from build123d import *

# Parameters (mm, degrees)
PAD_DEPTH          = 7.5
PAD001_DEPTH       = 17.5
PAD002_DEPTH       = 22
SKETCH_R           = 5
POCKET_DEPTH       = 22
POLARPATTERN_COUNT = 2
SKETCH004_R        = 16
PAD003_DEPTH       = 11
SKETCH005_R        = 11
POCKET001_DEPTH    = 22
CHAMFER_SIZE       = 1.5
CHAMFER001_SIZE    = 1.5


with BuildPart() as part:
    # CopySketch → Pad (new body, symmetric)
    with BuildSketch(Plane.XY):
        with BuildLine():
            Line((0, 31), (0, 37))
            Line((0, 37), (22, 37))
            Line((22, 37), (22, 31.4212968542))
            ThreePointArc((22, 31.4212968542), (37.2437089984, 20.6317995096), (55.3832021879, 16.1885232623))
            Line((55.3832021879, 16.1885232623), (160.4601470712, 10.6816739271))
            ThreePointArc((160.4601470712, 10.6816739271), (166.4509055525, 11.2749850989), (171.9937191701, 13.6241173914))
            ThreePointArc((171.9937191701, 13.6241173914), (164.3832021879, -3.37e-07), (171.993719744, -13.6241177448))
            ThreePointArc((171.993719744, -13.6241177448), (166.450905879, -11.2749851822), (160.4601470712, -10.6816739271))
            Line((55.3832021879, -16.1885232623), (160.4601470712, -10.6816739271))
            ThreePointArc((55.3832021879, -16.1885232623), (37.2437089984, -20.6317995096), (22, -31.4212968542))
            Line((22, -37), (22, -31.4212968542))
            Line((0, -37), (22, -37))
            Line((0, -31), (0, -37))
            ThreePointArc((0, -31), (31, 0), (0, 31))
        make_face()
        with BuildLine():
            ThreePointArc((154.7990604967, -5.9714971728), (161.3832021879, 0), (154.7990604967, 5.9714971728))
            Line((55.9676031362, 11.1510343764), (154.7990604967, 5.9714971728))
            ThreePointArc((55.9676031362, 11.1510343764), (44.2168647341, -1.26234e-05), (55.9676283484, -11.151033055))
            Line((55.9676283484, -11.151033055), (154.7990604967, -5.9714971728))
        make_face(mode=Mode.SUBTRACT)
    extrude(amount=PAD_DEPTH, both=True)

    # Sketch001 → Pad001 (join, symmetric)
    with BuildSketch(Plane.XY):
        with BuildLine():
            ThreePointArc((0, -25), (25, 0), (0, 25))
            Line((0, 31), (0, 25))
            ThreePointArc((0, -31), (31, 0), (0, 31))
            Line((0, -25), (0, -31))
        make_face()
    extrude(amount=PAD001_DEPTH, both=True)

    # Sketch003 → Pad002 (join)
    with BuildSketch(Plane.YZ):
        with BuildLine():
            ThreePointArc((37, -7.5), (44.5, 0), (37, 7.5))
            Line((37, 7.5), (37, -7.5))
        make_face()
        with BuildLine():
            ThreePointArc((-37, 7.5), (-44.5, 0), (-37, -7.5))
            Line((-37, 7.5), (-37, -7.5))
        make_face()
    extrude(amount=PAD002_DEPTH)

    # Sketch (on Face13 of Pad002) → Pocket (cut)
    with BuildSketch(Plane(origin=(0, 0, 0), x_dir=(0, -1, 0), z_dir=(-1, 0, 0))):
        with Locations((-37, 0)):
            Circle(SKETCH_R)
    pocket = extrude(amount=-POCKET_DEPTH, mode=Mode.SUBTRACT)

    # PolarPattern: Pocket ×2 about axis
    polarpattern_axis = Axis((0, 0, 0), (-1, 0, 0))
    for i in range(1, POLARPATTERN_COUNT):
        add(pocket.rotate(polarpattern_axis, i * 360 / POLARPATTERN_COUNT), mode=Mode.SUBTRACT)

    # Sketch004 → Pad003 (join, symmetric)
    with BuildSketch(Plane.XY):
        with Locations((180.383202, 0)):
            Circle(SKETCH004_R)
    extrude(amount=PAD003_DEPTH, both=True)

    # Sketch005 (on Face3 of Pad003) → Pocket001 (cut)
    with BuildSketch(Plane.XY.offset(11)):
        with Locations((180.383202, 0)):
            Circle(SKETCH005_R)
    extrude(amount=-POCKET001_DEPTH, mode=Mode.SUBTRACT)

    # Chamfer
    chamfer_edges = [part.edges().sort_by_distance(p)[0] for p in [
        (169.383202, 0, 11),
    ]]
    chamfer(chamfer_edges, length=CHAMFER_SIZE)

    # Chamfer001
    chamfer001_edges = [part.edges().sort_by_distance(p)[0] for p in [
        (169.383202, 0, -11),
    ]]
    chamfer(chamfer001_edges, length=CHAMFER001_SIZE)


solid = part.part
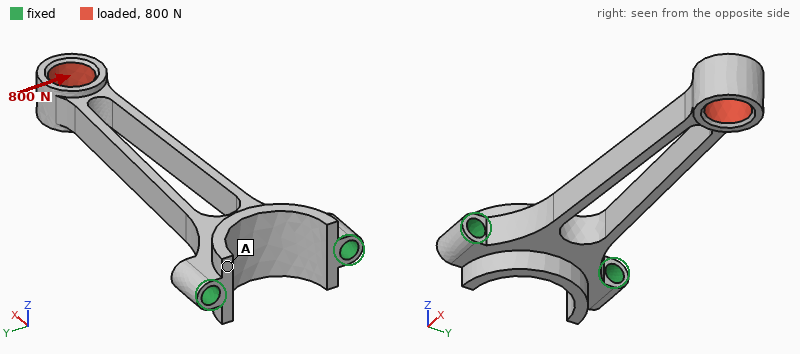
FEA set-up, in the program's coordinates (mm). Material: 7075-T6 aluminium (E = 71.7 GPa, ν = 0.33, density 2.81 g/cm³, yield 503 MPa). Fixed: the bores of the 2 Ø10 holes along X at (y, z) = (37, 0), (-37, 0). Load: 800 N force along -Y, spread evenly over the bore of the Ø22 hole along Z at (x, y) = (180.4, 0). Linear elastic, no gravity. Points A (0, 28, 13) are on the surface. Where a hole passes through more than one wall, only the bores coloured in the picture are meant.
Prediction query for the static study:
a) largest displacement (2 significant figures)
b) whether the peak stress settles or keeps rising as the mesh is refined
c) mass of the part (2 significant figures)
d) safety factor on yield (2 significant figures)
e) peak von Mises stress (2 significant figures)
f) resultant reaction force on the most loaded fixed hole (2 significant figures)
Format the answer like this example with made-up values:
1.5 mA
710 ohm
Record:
2.3 mm
settles
180 g
1.8
280 MPa
2.6 kN
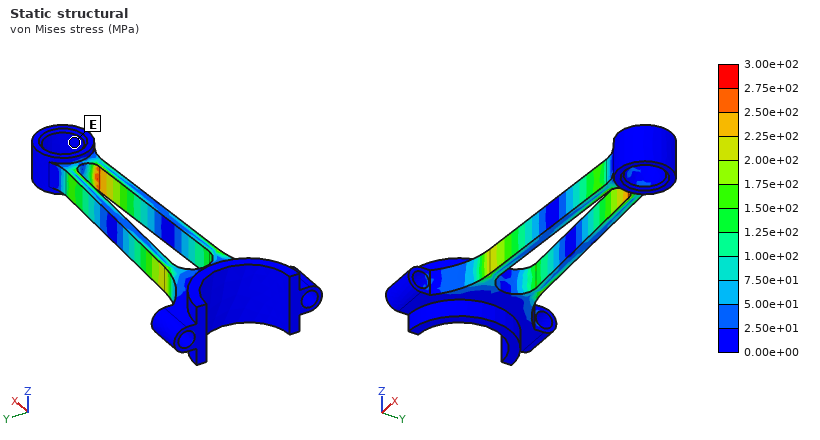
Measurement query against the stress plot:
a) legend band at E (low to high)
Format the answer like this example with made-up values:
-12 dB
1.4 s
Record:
0.00e+00 to 2.50e+01 MPa
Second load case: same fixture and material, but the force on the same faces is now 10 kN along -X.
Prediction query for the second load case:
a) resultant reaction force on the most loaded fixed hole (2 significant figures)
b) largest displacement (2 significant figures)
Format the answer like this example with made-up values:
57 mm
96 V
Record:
6.0 kN
0.17 mm
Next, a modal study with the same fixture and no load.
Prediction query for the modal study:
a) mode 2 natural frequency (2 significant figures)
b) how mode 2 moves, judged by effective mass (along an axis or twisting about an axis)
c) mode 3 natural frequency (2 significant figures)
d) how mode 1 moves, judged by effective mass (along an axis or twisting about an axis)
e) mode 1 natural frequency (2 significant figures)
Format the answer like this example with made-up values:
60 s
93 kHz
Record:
410 Hz
along Y
1400 Hz
along Z
360 Hz
